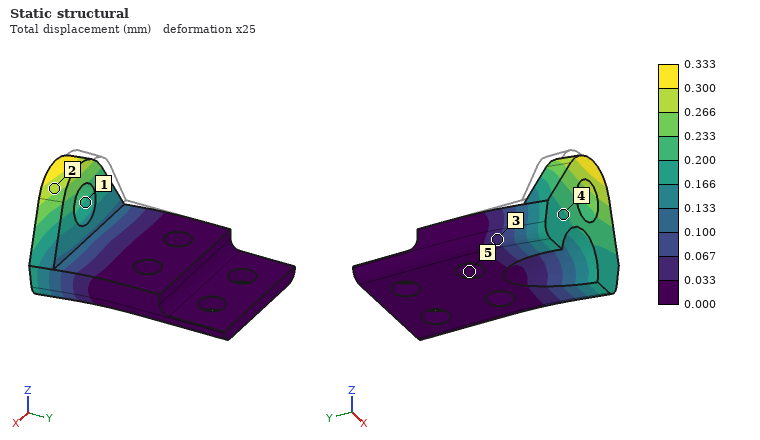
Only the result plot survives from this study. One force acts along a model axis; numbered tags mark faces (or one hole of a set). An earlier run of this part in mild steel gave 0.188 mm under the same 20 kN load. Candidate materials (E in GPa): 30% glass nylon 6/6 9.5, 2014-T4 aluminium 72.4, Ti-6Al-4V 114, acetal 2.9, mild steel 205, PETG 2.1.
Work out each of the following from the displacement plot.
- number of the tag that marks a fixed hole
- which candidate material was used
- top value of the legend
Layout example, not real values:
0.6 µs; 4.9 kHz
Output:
5; Ti-6Al-4V; 0.333 mm
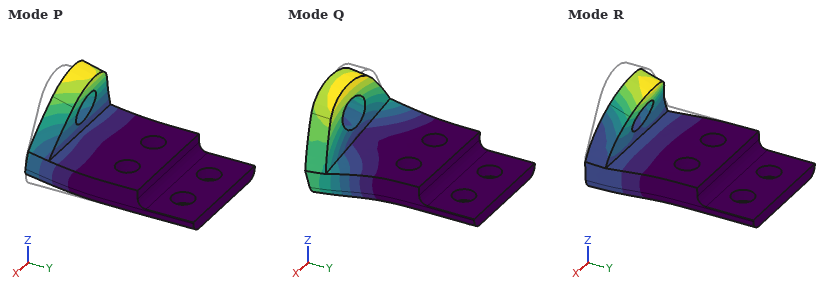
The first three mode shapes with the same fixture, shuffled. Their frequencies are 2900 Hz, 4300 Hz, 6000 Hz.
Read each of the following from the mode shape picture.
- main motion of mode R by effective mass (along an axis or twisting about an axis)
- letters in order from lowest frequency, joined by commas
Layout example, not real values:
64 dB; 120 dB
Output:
along Z; P, Q, R
